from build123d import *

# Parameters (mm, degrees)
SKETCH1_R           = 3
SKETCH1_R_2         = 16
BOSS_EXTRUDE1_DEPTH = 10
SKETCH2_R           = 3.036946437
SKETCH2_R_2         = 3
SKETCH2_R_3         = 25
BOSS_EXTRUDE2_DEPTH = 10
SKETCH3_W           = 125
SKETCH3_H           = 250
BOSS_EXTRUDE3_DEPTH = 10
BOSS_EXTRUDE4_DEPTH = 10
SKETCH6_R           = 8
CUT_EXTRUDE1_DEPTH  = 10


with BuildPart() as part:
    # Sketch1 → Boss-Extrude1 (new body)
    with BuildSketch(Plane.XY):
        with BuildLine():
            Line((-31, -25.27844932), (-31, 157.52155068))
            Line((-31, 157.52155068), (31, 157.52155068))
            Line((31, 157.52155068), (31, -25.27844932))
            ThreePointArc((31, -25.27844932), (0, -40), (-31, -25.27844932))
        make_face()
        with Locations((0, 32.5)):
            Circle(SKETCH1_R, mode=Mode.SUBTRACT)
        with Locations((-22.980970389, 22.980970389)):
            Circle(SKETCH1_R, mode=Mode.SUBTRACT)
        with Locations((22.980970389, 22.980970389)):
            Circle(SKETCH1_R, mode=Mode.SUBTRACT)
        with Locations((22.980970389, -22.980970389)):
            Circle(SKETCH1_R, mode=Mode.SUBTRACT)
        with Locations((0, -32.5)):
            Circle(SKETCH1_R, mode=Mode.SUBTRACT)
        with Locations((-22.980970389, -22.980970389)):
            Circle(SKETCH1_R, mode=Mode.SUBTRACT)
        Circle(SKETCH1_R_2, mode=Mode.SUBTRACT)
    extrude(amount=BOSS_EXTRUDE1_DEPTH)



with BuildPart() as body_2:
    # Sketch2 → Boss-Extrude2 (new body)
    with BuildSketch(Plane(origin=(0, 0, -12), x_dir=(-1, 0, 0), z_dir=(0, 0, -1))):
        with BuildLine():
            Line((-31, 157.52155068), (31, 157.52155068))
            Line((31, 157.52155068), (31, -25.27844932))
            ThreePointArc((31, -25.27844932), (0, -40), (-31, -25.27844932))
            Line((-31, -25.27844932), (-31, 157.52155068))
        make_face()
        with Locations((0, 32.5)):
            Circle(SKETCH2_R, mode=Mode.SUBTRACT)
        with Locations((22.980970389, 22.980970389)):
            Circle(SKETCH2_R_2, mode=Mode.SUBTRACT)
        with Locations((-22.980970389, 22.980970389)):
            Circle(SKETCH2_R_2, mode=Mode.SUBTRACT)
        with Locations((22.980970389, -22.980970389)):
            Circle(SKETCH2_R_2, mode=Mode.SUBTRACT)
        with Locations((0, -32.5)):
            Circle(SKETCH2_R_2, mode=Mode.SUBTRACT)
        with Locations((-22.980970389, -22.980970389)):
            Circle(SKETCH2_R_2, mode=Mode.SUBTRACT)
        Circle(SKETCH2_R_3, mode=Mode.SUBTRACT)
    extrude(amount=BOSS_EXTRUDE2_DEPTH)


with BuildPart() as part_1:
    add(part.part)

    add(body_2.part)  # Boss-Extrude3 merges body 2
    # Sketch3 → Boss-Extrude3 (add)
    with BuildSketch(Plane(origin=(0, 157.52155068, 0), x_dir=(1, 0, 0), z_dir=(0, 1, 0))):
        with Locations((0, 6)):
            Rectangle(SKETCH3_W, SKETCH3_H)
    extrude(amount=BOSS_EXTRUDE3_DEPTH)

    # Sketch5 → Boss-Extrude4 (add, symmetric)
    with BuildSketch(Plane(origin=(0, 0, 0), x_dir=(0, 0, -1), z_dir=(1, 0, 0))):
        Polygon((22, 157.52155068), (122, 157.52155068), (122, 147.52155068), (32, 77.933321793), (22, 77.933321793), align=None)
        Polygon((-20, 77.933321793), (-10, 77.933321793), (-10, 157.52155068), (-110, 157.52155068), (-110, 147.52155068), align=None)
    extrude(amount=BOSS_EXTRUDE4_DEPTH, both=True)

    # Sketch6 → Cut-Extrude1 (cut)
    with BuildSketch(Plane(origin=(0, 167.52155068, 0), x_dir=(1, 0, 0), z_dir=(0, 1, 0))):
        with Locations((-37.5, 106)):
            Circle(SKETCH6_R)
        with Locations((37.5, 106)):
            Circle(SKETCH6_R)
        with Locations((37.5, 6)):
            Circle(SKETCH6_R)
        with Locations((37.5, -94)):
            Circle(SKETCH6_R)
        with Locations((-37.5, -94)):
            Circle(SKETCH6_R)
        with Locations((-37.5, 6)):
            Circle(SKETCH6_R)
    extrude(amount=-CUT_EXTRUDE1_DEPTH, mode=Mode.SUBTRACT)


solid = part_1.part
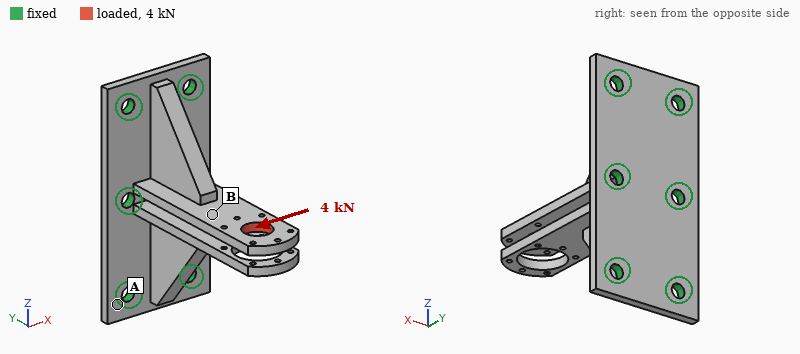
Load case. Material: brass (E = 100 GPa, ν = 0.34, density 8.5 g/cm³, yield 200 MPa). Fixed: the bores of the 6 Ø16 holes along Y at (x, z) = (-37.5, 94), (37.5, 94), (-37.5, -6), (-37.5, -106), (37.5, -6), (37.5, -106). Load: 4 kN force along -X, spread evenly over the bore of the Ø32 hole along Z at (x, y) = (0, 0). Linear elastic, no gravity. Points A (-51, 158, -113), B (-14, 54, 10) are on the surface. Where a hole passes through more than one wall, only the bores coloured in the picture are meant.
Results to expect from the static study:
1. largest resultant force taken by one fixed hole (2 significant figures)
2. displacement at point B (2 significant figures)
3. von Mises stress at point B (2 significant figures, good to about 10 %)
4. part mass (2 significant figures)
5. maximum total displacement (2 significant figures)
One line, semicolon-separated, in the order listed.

9.6 kN; 0.19 mm; 18 MPa; 6.0 kg; 0.47 mm
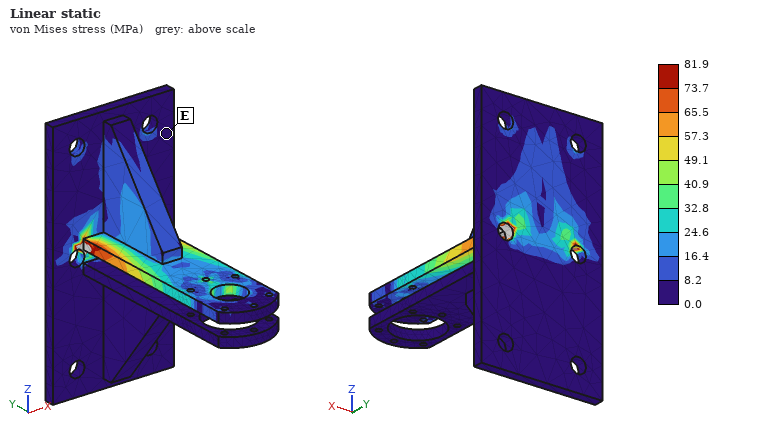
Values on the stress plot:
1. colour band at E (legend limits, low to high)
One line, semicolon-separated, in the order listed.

0.0 to 8.2 MPa
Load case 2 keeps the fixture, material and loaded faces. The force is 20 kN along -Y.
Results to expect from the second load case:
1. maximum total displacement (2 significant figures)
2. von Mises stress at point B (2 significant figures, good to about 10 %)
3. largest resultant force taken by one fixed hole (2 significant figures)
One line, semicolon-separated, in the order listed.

0.15 mm; 32 MPa; 10 kN
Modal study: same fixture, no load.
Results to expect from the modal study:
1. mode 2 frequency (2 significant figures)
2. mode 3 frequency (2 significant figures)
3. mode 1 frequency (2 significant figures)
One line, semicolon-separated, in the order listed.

440 Hz; 850 Hz; 390 Hz
